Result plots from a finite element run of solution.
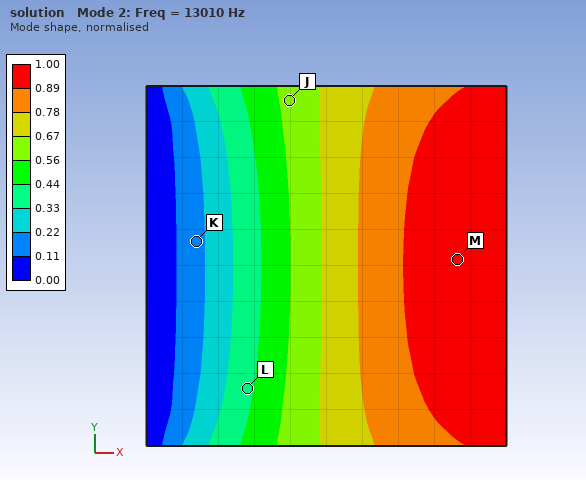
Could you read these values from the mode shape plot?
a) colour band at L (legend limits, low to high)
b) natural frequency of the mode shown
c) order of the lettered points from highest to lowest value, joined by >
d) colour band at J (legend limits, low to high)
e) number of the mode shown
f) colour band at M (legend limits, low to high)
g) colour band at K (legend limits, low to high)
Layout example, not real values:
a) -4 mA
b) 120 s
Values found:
a) 0.33 to 0.44
b) 13010 Hz
c) M > J > L > K
d) 0.56 to 0.67
e) 2
f) 0.89 to 1.00
g) 0.11 to 0.22
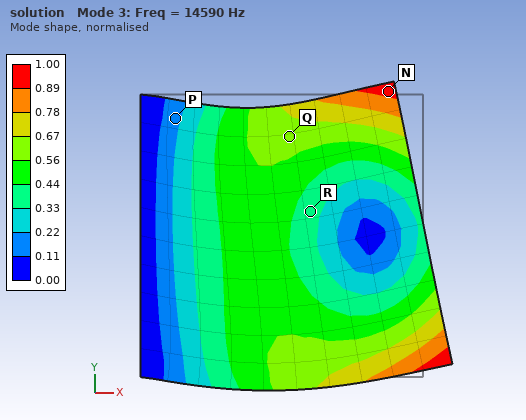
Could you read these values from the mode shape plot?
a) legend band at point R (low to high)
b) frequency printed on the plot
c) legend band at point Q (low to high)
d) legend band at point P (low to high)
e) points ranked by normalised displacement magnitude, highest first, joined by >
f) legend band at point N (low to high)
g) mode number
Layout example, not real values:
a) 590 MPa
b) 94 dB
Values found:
a) 0.33 to 0.44
b) 14590 Hz
c) 0.56 to 0.67
d) 0.11 to 0.22
e) N > Q > R > P
f) 0.89 to 1.00
g) 3
